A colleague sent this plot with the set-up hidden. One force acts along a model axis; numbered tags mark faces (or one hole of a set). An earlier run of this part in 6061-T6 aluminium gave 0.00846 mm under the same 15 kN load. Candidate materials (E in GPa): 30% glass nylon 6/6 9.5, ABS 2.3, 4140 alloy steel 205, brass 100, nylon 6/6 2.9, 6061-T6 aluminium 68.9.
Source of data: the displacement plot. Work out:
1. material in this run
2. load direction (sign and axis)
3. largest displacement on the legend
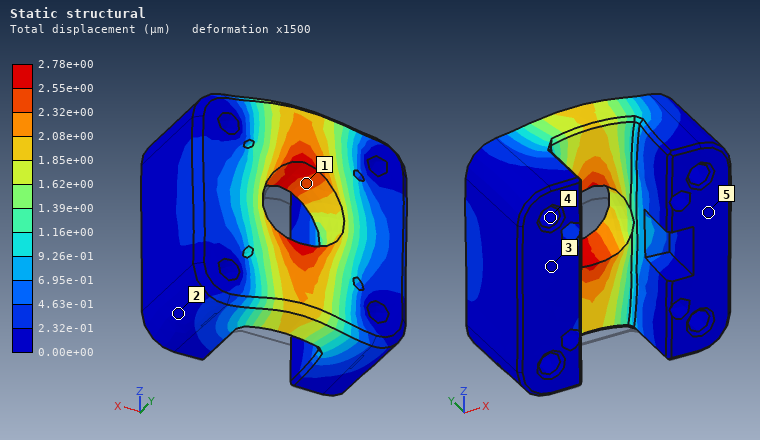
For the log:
4140 alloy steel
+Z
2.78e+00 µm
